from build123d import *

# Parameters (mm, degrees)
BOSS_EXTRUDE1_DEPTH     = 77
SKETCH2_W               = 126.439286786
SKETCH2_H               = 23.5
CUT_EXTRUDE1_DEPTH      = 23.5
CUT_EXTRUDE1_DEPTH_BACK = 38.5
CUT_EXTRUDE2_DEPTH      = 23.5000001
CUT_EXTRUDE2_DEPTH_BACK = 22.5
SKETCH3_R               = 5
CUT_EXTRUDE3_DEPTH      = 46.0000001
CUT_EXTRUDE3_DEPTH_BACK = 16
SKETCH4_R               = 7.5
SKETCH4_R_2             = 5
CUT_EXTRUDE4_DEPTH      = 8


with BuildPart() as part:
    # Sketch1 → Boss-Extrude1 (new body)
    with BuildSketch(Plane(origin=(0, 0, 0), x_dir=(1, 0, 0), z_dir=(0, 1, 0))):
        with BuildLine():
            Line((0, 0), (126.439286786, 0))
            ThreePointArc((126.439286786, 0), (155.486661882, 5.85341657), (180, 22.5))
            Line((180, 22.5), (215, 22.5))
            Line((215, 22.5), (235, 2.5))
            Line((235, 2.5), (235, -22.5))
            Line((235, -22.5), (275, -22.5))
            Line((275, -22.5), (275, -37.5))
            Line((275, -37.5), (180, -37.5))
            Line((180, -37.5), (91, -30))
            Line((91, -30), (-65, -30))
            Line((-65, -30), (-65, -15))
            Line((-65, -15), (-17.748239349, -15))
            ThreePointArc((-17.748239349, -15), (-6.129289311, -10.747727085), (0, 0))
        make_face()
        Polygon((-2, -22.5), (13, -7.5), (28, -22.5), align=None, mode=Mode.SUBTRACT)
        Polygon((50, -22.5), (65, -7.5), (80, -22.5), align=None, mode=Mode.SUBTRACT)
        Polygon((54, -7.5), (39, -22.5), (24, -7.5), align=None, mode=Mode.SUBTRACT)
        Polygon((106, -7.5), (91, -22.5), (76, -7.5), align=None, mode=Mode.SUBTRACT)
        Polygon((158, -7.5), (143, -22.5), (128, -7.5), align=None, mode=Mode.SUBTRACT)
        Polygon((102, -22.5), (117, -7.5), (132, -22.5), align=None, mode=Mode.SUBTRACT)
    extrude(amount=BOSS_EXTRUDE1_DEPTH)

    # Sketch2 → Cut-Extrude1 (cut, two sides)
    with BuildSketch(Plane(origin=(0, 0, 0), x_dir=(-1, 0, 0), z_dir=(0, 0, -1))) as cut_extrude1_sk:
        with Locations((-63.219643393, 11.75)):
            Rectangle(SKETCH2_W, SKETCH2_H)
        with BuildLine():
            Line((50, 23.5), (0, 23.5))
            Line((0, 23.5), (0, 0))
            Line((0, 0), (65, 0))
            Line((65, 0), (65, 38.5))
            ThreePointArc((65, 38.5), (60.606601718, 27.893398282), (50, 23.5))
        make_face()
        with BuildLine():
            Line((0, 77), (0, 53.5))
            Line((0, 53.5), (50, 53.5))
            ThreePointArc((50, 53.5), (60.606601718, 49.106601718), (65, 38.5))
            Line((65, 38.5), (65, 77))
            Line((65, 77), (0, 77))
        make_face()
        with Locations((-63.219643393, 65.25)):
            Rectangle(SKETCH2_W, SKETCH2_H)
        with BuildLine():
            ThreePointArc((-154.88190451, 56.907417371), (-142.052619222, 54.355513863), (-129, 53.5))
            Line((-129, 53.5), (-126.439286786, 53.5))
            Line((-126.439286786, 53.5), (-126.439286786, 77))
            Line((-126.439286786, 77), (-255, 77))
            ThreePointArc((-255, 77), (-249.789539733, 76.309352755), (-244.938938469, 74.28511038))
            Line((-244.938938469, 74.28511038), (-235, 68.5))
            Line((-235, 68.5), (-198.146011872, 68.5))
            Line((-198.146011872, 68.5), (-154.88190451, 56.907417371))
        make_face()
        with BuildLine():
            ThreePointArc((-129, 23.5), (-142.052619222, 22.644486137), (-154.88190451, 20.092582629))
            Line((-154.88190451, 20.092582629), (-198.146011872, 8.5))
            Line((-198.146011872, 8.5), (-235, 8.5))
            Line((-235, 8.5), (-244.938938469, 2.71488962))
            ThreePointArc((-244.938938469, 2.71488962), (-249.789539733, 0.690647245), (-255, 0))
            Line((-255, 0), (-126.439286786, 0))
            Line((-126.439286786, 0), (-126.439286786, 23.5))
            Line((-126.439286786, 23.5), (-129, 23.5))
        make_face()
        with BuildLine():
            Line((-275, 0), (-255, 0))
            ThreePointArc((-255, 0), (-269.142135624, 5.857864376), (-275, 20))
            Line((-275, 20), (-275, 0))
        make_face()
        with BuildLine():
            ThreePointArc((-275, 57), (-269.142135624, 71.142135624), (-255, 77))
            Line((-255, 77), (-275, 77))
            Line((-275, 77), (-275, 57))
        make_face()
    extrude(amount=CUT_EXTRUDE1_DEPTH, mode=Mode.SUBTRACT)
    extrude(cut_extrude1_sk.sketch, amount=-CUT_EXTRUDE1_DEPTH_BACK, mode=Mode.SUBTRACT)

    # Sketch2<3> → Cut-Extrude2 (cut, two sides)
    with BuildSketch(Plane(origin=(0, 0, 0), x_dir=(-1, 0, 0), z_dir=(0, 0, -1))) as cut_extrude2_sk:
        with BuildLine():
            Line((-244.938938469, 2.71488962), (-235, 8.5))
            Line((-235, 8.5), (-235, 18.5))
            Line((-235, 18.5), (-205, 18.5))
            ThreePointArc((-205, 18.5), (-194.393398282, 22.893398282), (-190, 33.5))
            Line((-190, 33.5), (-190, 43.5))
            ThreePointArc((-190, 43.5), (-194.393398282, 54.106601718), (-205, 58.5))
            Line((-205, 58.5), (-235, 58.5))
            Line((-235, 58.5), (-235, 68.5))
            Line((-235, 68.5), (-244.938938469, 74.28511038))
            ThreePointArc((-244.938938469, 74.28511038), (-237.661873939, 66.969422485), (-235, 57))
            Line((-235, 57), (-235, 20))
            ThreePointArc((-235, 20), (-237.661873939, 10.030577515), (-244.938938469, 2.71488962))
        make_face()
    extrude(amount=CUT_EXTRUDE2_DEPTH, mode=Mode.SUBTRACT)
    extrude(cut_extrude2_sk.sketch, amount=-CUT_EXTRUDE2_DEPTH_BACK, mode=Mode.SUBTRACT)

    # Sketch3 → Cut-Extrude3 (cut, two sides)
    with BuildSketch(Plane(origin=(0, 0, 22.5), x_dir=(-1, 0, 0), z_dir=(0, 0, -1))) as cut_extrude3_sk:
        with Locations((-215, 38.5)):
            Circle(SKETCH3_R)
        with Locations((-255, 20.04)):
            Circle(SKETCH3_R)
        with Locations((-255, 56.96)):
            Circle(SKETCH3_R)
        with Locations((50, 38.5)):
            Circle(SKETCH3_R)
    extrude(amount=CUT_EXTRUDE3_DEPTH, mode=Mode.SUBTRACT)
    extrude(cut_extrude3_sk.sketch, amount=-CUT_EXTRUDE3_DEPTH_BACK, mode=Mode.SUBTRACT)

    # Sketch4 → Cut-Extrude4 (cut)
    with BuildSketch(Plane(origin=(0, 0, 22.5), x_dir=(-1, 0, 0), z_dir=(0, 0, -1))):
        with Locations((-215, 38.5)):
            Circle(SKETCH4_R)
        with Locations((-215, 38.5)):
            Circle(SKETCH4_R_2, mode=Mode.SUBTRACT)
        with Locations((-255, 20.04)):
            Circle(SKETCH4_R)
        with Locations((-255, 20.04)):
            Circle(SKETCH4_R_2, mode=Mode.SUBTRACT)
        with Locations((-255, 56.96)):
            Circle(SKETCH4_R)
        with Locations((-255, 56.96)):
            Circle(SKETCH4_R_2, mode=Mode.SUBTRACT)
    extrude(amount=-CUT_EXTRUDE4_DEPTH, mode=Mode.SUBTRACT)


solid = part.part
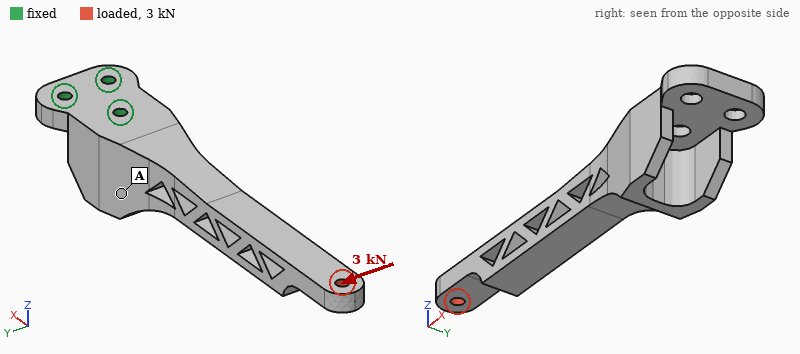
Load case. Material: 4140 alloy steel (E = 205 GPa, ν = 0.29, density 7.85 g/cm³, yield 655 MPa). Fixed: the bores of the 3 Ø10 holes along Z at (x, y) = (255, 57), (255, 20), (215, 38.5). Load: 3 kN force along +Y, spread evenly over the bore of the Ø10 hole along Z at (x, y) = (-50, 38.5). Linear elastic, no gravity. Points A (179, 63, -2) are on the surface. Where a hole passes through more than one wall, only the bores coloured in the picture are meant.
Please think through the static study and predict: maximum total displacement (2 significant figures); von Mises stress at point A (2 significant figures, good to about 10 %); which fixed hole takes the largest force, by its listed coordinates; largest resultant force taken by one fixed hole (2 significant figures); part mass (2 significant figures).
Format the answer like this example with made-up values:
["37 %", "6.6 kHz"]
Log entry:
["1.3 mm", "29 MPa", "(215, 38.5)", "13 kN", "2.7 kg"]
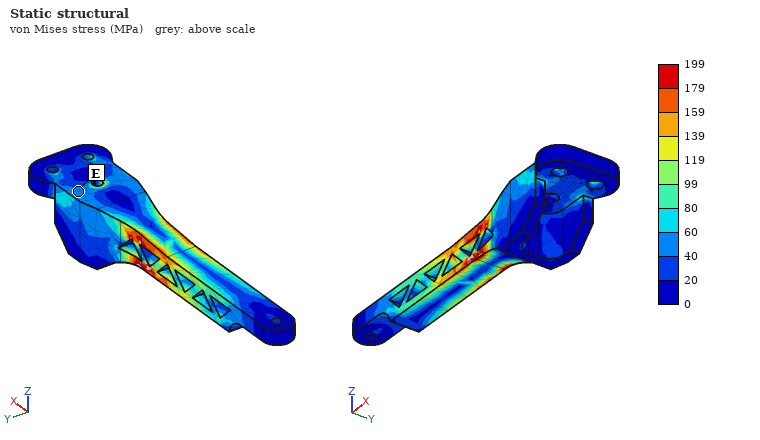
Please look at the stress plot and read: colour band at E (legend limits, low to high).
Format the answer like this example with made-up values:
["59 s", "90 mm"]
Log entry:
["40 to 60 MPa"]
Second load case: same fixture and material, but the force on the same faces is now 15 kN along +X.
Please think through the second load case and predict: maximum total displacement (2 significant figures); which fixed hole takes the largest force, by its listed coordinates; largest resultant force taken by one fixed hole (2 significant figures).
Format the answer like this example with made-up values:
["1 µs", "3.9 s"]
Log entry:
["0.10 mm", "(215, 38.5)", "7.6 kN"]
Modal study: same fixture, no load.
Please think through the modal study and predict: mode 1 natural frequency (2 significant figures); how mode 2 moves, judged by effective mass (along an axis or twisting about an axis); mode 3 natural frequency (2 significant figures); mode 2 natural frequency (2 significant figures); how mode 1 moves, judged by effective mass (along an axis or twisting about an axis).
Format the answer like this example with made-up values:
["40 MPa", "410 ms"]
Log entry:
["440 Hz", "along Y", "1800 Hz", "490 Hz", "along Z"]
